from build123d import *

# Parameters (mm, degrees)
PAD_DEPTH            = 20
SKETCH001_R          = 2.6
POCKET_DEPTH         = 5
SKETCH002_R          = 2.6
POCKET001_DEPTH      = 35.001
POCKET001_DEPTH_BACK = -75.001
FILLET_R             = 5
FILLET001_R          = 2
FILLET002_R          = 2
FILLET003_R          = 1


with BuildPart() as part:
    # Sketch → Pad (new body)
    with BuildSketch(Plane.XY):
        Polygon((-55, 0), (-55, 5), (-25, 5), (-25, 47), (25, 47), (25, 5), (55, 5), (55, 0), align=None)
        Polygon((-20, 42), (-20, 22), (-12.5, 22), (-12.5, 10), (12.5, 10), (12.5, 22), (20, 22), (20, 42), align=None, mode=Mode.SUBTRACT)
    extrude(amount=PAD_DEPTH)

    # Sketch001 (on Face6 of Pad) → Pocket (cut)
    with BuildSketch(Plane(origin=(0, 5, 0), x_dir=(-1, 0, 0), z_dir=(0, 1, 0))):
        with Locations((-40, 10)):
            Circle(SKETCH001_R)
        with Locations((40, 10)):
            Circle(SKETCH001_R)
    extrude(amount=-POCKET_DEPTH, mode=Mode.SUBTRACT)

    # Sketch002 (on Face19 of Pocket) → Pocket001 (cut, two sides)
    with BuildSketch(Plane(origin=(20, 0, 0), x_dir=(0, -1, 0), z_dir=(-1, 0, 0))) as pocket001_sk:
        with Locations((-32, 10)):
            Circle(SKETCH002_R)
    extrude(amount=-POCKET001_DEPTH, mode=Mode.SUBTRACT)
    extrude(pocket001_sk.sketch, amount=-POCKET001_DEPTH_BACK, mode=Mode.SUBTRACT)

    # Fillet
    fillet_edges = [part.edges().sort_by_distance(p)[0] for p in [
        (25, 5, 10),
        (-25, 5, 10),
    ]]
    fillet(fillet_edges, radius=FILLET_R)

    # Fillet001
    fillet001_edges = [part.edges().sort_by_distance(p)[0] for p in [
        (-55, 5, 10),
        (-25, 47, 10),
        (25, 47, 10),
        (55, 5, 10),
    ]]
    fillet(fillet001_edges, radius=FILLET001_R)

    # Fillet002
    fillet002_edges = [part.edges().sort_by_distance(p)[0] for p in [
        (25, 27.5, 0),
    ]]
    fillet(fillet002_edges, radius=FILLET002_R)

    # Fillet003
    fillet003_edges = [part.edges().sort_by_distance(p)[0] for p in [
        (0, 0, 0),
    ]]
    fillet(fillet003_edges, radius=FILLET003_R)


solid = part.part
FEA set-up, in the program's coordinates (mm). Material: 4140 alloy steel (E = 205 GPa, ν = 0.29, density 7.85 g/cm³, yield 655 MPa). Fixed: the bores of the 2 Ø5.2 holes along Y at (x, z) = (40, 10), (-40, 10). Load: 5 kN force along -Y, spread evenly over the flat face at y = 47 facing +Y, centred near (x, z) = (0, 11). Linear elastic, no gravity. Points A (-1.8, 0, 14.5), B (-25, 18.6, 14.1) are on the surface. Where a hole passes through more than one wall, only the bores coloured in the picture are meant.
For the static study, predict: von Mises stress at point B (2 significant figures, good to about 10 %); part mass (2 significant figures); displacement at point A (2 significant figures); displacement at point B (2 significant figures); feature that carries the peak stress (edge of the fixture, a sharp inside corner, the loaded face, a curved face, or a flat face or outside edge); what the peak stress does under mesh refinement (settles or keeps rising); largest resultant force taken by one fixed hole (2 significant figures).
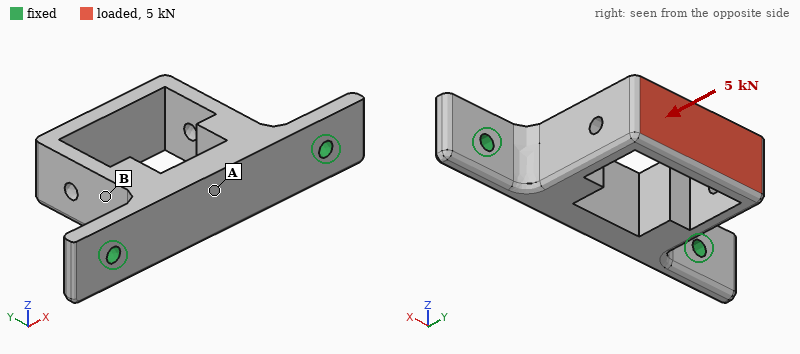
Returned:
61 MPa
240 g
26 µm
27 µm
edge of the fixture
keeps rising
2.8 kN
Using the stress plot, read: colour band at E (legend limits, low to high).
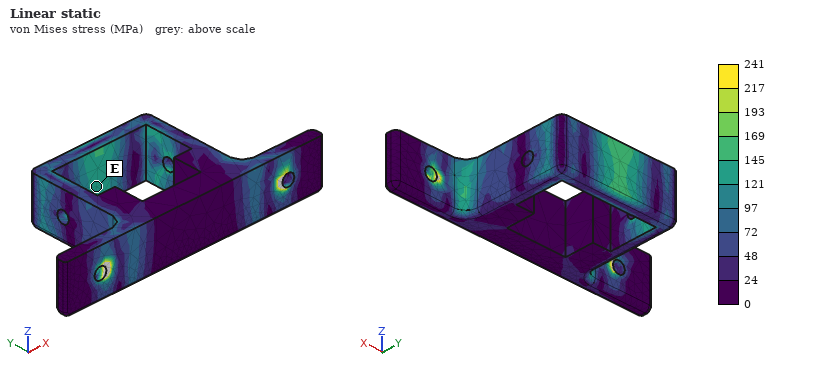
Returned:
121 to 145 MPa
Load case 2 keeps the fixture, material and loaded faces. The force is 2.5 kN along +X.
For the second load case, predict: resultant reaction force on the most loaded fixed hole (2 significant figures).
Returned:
2.1 kN
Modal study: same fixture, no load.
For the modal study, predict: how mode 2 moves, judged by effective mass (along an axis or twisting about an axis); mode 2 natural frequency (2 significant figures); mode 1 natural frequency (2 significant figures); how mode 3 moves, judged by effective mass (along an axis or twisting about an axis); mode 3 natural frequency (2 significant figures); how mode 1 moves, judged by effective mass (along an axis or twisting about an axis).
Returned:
along X
3600 Hz
1500 Hz
along Y
4400 Hz
along Z
